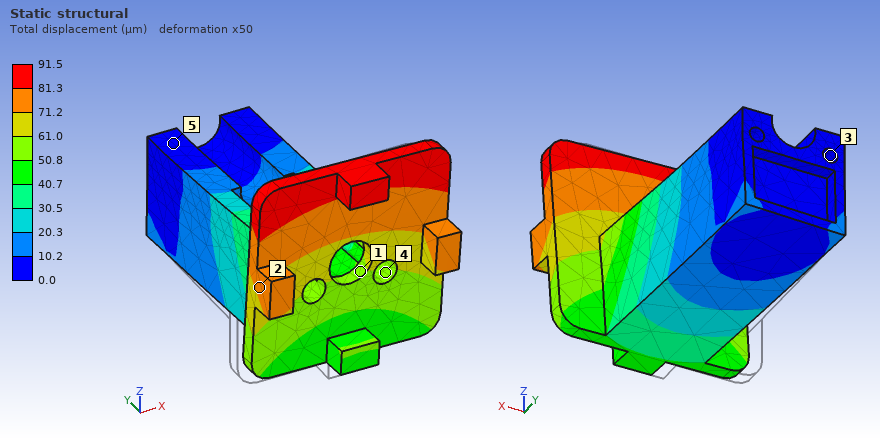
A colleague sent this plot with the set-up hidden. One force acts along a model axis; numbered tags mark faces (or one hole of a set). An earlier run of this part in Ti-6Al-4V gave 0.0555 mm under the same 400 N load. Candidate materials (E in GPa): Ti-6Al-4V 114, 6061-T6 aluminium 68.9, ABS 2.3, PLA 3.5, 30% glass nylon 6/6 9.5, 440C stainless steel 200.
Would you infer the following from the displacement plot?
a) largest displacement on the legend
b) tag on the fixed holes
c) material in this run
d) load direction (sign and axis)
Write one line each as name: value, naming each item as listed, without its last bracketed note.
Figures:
largest displacement on the legend: 91.5 µm
tag on the fixed holes: 3
material in this run: 6061-T6 aluminium
load direction: +X
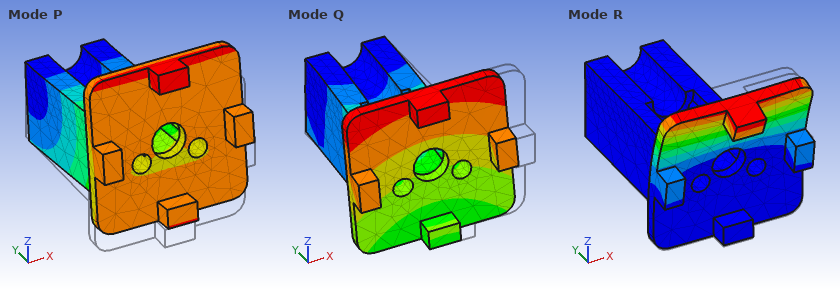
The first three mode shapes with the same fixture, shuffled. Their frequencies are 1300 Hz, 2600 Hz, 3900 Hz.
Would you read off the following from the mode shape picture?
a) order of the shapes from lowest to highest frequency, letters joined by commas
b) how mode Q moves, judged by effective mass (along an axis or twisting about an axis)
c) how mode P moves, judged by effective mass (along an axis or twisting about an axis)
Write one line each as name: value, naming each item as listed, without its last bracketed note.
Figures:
order of the shapes from lowest to highest frequency, letters joined by commas: P, Q, R
how mode Q moves, judged by effective mass: along X
how mode P moves, judged by effective mass: along Z
